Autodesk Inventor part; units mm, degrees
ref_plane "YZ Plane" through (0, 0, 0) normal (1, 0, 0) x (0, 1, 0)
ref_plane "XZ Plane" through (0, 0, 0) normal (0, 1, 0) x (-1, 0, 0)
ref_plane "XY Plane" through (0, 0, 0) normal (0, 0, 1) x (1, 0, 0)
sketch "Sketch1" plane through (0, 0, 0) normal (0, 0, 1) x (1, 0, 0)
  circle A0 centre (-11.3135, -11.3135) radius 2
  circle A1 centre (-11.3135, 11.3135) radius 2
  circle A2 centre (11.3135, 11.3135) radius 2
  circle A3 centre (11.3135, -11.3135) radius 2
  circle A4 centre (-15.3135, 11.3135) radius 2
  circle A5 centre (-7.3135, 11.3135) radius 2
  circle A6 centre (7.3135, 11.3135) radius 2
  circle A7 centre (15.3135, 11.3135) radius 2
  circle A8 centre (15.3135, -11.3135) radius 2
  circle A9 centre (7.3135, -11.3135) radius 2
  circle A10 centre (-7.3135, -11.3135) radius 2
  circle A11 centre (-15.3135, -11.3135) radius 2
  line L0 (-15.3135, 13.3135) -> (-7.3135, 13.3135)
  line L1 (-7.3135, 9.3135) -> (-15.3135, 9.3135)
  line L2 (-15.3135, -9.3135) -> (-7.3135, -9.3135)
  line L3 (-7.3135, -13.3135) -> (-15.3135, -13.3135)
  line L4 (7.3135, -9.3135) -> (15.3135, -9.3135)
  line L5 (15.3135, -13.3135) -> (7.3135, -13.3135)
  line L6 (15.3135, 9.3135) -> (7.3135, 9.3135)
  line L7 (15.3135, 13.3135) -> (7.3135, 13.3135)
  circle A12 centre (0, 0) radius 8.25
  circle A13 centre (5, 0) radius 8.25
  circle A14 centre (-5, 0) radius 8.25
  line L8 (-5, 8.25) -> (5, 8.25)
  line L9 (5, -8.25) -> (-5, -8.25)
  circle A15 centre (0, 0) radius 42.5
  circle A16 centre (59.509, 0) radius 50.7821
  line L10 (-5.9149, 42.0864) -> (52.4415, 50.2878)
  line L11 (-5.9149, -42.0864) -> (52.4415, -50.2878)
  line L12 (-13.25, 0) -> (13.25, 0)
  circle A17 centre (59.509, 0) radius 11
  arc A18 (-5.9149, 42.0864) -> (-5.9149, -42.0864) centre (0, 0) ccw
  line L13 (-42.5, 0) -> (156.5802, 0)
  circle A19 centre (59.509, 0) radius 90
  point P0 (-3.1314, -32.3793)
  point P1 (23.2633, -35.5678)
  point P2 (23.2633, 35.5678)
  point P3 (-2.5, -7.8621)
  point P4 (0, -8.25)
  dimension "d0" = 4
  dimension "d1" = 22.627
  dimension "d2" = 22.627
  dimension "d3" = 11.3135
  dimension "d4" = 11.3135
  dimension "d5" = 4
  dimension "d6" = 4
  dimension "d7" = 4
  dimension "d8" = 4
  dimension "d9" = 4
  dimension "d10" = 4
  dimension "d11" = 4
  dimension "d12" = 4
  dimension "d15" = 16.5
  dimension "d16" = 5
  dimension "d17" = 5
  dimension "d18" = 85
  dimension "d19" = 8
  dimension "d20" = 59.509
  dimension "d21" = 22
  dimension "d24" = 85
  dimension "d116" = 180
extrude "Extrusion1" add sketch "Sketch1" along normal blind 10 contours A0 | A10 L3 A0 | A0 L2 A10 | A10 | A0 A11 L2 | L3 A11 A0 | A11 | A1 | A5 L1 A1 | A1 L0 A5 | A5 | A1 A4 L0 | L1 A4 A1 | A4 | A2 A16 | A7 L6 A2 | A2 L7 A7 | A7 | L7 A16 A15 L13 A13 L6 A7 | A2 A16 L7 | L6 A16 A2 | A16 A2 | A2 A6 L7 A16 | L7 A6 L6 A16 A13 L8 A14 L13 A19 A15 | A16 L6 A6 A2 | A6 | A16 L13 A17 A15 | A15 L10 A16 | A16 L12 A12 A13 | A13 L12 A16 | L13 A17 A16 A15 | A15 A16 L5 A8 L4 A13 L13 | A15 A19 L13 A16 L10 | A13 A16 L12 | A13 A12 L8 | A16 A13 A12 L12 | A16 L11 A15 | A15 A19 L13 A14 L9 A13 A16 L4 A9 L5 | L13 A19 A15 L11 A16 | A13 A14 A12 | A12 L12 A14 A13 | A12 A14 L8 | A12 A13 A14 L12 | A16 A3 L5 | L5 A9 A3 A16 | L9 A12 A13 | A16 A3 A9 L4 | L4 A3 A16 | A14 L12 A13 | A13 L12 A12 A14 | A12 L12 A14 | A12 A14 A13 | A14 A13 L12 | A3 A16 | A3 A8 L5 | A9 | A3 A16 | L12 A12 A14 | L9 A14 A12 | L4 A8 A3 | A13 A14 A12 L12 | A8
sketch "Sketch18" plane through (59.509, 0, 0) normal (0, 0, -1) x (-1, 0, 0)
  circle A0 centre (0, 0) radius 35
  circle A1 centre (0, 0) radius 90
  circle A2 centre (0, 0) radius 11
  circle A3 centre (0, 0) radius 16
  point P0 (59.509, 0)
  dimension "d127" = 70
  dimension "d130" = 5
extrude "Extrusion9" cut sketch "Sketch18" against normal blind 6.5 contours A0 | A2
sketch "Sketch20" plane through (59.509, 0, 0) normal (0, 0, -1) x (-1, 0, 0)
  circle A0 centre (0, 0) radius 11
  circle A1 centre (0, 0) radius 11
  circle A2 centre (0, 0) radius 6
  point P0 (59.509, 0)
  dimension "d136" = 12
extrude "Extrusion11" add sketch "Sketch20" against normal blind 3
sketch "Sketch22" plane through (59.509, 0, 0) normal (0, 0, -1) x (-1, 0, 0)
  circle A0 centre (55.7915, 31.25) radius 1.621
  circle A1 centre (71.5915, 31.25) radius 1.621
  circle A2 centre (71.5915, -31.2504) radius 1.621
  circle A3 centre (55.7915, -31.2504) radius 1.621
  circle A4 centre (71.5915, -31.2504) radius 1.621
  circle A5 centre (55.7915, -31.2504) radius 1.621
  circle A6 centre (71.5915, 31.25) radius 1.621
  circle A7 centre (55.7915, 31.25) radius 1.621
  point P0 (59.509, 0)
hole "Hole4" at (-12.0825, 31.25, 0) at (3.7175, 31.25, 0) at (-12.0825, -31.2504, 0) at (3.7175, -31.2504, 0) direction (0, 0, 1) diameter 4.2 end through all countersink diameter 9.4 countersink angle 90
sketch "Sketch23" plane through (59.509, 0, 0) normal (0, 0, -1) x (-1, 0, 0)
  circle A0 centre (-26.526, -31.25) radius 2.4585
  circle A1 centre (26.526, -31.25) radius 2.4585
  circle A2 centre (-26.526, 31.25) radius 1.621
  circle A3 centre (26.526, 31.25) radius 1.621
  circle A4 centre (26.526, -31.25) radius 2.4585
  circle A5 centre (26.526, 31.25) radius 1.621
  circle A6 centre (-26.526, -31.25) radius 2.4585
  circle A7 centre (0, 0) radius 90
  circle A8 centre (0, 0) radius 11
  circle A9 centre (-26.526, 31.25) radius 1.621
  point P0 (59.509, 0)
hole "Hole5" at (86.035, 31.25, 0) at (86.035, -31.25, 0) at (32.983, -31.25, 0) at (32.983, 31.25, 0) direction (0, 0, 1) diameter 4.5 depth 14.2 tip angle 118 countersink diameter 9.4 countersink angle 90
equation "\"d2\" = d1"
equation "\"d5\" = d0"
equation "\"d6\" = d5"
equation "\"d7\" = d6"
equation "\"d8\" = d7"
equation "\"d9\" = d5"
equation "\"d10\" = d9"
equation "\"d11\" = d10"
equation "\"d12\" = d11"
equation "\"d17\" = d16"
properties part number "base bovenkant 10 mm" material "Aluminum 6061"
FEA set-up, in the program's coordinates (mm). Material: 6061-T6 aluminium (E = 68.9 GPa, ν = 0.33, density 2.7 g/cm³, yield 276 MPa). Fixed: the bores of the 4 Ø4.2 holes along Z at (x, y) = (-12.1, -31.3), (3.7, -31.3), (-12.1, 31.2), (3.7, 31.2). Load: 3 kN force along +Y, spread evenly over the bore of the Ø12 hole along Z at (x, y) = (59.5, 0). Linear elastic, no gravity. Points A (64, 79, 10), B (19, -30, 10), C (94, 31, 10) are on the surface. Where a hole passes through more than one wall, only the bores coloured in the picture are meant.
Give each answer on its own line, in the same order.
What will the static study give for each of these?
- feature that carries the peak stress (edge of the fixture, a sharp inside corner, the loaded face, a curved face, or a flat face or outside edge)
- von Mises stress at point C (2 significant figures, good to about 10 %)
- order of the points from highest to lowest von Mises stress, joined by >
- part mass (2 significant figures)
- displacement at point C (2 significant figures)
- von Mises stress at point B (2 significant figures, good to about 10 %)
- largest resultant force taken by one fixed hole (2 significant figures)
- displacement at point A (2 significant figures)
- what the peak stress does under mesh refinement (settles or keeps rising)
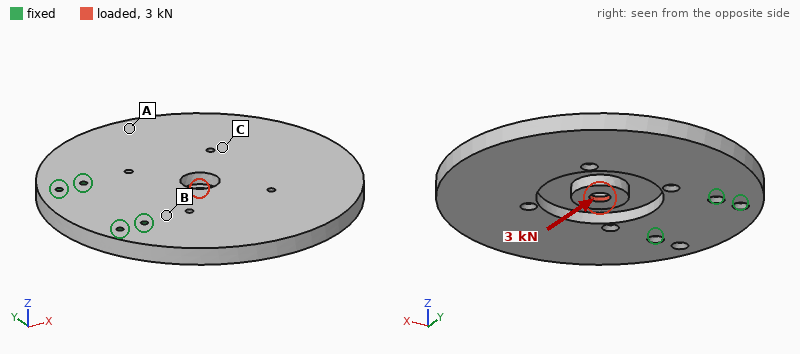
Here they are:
edge of the fixture
6.7 MPa
B > C > A
620 g
32 µm
12 MPa
2.4 kN
35 µm
keeps rising
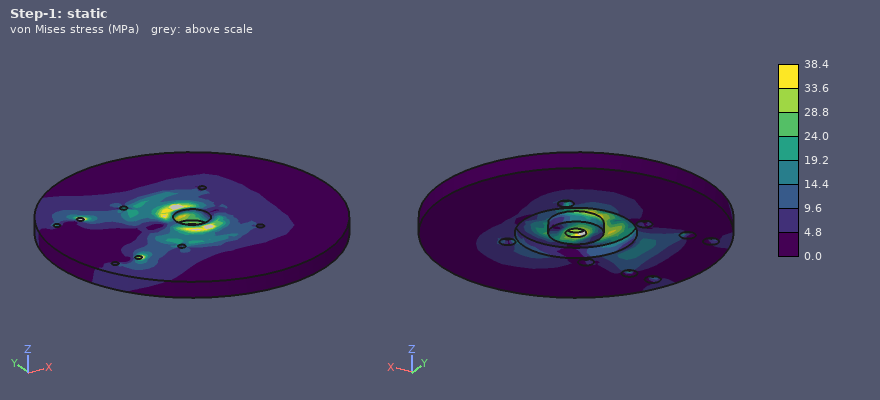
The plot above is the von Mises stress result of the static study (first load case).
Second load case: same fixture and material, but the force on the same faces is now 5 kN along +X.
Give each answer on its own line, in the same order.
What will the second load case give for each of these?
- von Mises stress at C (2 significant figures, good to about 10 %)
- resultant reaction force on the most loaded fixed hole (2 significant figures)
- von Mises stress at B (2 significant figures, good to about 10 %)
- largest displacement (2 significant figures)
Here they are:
11 MPa
1.6 kN
13 MPa
0.29 mm
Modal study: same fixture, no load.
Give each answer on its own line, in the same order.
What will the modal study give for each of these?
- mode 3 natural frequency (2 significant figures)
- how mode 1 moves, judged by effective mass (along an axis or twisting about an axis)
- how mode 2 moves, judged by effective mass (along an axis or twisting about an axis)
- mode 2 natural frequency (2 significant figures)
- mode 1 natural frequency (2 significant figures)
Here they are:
1600 Hz
along Z
twisting about X
750 Hz
360 Hz
